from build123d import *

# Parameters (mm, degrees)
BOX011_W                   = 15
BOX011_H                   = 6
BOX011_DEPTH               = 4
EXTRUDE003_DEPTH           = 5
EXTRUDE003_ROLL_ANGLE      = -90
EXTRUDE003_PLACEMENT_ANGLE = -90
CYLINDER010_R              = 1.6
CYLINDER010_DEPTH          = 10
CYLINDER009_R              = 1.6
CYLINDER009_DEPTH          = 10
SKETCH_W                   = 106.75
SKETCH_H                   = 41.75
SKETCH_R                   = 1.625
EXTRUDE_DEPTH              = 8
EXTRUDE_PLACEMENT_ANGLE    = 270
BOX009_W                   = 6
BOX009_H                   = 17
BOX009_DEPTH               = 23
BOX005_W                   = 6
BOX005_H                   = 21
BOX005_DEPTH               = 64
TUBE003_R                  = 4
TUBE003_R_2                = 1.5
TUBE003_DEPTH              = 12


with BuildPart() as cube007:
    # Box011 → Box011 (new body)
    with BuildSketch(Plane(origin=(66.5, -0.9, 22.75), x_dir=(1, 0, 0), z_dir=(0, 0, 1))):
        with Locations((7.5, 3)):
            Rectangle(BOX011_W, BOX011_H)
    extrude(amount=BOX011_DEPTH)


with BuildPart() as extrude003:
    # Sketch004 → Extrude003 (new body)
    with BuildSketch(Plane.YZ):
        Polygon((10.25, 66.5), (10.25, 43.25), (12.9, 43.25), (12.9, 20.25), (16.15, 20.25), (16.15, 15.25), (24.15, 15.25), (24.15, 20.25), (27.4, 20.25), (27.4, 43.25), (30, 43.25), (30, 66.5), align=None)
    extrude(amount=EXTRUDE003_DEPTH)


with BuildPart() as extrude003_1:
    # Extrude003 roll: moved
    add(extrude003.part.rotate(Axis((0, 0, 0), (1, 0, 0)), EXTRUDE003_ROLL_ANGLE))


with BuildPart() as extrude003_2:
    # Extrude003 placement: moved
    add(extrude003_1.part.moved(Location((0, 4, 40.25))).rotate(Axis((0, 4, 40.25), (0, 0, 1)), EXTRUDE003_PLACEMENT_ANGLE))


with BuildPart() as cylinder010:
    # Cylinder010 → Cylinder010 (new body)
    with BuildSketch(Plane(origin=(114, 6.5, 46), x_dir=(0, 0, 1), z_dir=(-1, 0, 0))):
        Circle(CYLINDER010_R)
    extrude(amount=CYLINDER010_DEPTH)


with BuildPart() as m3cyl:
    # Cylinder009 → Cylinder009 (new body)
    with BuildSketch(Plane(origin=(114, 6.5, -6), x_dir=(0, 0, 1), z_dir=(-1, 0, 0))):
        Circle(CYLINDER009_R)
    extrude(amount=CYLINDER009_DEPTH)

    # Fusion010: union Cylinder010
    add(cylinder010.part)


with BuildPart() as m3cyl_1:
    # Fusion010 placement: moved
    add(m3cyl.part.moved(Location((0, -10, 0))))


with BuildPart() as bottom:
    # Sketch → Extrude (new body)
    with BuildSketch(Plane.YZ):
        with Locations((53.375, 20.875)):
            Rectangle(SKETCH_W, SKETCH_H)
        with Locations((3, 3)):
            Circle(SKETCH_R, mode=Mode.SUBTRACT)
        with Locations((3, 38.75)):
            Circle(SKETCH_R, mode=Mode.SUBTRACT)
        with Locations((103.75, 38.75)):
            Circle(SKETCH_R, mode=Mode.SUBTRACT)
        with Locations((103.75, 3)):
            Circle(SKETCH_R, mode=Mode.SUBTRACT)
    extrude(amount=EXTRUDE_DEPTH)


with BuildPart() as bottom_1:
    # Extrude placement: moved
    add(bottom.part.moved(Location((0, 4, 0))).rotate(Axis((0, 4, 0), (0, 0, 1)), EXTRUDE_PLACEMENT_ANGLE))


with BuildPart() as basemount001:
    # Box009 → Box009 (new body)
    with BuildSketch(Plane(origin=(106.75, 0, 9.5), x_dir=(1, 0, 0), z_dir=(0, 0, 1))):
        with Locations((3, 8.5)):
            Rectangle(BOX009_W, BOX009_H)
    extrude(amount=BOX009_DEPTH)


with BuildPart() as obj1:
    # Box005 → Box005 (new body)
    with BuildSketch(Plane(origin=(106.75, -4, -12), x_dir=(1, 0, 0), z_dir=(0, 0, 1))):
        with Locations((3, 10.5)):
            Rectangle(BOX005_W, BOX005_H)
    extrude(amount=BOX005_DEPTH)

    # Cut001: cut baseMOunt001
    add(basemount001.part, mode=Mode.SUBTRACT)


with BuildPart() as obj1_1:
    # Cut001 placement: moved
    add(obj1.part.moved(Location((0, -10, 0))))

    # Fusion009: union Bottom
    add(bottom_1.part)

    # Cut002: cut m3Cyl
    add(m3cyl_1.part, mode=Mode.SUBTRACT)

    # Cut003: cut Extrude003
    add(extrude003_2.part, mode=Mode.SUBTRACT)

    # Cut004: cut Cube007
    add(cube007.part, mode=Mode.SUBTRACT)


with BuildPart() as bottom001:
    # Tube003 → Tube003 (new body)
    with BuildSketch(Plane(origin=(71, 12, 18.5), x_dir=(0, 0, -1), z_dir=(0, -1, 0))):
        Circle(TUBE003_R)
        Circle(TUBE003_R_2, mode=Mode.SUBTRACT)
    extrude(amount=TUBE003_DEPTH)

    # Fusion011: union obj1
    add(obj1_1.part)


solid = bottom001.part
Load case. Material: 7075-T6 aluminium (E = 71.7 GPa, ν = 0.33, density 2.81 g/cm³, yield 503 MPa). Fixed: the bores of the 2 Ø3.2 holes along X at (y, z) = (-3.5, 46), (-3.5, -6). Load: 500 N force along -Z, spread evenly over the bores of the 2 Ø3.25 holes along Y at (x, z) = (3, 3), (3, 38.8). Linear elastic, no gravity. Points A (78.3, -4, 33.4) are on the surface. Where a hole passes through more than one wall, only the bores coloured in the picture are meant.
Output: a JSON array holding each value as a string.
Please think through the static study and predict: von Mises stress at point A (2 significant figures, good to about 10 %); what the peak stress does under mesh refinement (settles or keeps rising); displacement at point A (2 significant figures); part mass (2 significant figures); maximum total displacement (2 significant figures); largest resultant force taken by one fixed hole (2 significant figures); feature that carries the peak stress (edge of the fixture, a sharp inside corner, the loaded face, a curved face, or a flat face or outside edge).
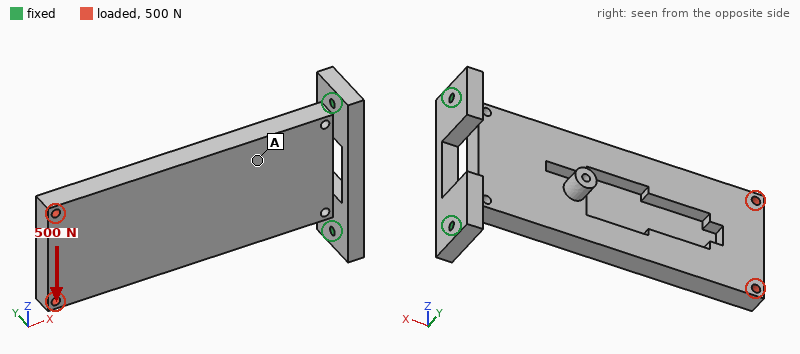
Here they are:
["12 MPa", "keeps rising", "0.031 mm", "100 g", "0.16 mm", "1.2 kN", "edge of the fixture"]
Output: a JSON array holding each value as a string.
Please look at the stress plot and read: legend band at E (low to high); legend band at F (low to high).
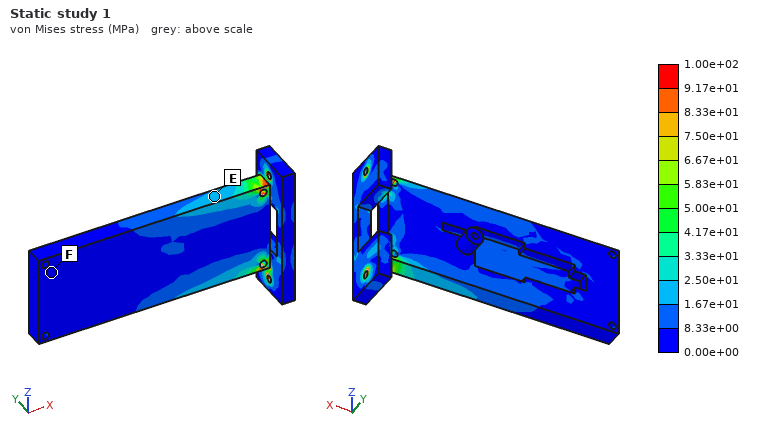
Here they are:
["1.67e+01 to 2.50e+01 MPa", "0.00e+00 to 8.33e+00 MPa"]
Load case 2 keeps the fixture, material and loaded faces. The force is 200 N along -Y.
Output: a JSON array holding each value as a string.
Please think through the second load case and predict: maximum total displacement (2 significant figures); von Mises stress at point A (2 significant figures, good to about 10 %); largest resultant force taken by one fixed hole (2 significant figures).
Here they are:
["1.3 mm", "36 MPa", "130 N"]
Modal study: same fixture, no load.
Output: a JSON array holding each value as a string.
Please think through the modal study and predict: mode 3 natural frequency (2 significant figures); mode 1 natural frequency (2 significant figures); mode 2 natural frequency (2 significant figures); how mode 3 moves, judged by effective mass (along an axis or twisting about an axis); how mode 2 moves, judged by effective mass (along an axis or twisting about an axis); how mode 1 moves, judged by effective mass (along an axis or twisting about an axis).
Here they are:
["2200 Hz", "380 Hz", "1700 Hz", "twisting about X", "along Z", "along Y"]
